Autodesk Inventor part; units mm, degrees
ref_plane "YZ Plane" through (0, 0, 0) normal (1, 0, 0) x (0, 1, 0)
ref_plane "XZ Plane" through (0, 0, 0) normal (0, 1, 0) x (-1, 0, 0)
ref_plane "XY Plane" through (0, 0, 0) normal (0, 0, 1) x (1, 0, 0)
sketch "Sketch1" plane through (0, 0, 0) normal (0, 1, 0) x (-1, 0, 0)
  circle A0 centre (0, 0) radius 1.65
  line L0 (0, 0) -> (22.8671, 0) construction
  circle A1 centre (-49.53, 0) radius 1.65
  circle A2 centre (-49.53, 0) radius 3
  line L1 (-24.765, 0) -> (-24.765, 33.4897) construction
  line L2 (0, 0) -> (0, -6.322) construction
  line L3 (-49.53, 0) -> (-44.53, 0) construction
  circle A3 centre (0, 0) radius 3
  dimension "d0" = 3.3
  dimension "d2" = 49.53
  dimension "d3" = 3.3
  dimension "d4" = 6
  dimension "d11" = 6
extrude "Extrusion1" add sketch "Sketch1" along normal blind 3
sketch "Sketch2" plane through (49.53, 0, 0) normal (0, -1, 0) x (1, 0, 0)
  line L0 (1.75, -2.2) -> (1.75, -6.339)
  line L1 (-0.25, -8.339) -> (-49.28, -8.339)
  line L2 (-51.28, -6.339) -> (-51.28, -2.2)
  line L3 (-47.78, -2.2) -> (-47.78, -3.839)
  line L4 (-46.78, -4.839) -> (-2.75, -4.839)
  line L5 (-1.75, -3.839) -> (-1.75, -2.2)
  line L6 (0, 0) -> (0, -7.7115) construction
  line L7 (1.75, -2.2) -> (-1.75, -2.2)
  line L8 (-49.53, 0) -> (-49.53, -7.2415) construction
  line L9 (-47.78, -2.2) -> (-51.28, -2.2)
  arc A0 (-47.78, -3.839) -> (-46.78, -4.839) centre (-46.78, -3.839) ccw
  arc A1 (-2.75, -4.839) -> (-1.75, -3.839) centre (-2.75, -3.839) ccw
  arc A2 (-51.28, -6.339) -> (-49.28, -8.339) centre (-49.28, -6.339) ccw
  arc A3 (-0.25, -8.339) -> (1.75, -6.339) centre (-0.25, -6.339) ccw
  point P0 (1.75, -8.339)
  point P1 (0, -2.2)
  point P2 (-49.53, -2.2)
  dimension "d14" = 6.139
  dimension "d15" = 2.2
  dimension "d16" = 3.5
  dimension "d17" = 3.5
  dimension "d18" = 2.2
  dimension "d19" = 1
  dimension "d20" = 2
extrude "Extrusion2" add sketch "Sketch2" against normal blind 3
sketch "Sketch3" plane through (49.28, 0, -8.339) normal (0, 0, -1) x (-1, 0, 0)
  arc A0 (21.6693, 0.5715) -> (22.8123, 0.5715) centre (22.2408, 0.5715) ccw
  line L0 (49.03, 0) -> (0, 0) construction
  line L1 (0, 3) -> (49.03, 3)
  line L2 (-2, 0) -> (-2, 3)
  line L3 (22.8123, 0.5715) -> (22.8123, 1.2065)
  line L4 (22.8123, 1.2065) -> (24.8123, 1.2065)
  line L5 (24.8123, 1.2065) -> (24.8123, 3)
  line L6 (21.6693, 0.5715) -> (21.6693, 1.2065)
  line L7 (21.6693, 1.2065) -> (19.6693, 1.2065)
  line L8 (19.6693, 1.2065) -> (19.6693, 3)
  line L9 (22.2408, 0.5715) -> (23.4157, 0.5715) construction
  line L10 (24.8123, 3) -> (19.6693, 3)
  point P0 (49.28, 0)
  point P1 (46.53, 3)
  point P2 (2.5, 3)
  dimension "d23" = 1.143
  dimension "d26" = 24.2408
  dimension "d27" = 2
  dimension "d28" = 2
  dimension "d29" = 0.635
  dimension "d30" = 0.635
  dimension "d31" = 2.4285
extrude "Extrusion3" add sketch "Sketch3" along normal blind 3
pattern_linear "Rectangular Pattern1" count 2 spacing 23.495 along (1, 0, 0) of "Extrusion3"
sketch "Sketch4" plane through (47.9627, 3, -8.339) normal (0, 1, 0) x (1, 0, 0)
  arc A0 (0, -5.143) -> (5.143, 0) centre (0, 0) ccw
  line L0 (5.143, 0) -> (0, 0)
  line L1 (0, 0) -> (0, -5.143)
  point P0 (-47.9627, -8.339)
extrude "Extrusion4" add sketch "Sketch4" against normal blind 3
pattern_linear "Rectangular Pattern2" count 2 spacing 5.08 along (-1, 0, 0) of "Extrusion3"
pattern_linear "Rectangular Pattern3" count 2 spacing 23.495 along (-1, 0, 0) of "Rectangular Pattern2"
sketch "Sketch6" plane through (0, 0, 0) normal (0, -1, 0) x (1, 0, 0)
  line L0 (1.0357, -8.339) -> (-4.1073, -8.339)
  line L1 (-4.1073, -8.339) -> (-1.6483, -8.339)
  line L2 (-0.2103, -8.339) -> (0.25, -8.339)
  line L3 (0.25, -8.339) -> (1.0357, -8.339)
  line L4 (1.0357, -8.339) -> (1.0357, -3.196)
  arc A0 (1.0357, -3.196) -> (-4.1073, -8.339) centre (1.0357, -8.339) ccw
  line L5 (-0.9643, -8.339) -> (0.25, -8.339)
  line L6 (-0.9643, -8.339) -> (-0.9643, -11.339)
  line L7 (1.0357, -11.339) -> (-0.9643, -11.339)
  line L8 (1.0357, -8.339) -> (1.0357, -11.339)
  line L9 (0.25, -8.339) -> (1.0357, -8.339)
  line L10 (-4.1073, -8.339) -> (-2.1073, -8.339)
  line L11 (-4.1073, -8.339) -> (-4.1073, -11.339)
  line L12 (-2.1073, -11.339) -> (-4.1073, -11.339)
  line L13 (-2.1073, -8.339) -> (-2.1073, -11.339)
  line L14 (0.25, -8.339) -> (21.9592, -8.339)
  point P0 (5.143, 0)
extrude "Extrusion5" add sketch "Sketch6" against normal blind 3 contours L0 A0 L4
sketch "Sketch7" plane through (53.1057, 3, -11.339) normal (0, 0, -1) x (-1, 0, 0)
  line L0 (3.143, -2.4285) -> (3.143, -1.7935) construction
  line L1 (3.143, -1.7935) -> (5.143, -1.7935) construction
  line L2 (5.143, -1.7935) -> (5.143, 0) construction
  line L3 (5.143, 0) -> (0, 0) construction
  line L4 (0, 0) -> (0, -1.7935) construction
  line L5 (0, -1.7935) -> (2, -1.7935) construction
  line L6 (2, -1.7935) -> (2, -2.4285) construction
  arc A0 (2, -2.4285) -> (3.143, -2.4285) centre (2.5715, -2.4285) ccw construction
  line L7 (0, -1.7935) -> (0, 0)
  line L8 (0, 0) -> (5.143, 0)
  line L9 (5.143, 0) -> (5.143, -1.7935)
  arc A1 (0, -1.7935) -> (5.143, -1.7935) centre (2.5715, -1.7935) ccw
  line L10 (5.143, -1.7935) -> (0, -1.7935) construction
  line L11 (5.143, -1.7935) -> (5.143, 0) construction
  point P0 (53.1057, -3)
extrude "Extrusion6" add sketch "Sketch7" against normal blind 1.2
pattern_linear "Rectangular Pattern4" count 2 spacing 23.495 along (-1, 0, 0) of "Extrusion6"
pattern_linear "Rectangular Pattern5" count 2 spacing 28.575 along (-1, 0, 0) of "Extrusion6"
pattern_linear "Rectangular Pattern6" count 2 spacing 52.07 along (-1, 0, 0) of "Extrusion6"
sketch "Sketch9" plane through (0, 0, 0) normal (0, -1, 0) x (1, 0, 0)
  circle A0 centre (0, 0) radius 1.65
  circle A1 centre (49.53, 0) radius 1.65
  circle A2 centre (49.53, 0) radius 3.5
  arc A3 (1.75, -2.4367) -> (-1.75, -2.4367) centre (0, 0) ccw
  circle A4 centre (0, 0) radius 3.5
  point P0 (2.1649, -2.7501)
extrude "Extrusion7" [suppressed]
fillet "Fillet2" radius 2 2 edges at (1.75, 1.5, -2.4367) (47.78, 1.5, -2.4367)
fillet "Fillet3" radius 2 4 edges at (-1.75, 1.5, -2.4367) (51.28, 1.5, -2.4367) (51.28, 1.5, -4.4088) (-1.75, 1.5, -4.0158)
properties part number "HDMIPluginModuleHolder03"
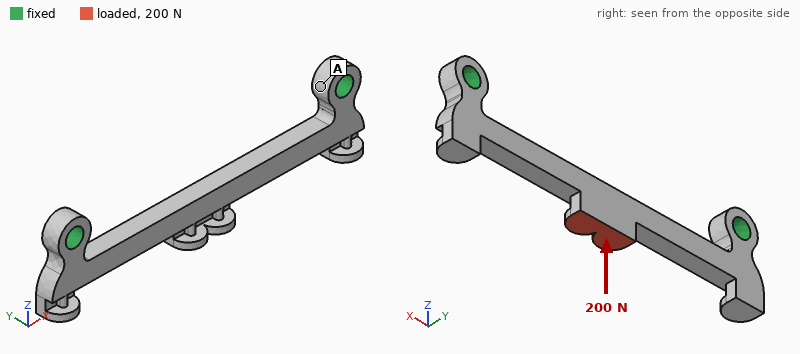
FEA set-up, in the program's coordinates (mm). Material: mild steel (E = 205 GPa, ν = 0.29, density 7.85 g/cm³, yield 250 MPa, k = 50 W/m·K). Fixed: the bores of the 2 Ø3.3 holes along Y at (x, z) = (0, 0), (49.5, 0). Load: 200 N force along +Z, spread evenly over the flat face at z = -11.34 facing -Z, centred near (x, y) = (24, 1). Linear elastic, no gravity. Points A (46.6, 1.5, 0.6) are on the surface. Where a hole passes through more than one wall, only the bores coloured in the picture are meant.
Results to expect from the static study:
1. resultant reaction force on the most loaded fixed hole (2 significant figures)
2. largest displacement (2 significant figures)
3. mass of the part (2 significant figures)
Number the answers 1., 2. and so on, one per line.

1. 210 N
2. 50 µm
3. 7.3 g
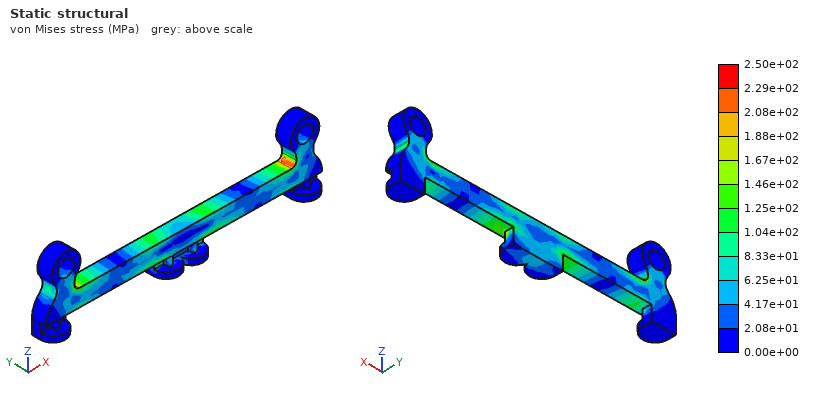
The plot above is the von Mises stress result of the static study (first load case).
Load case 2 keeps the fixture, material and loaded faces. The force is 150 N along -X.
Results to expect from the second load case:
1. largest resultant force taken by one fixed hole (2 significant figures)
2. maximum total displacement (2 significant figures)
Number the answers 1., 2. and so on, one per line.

1. 78 N
2. 5.6 µm
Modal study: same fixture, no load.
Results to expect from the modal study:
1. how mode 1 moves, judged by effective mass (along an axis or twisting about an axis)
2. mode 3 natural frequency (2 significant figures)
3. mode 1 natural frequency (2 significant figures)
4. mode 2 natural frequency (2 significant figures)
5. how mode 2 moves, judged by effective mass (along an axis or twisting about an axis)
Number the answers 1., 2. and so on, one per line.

1. along Y
2. 13 kHz
3. 4400 Hz
4. 6600 Hz
5. along Z
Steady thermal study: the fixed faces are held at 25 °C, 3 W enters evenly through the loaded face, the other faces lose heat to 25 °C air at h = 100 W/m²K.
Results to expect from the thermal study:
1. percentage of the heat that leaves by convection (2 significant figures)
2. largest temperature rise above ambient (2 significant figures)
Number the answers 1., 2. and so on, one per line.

1. 60 %
2. 48 K
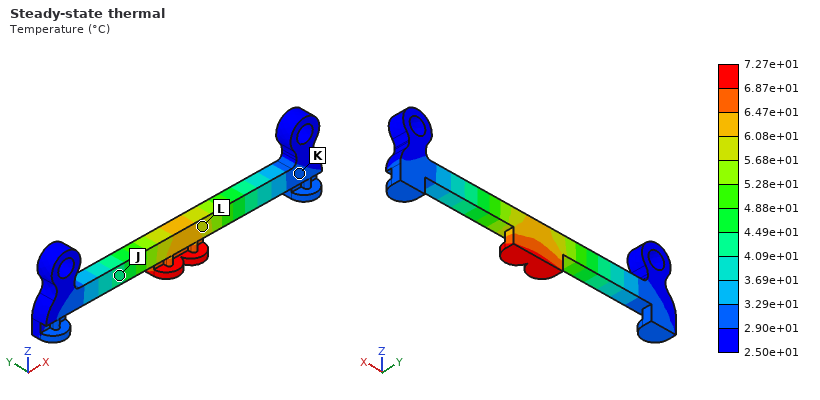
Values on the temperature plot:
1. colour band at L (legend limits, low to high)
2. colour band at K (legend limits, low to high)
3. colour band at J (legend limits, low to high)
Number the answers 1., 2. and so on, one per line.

1. 5.68e+01 to 6.08e+01 °C
2. 2.90e+01 to 3.29e+01 °C
3. 4.09e+01 to 4.49e+01 °C
